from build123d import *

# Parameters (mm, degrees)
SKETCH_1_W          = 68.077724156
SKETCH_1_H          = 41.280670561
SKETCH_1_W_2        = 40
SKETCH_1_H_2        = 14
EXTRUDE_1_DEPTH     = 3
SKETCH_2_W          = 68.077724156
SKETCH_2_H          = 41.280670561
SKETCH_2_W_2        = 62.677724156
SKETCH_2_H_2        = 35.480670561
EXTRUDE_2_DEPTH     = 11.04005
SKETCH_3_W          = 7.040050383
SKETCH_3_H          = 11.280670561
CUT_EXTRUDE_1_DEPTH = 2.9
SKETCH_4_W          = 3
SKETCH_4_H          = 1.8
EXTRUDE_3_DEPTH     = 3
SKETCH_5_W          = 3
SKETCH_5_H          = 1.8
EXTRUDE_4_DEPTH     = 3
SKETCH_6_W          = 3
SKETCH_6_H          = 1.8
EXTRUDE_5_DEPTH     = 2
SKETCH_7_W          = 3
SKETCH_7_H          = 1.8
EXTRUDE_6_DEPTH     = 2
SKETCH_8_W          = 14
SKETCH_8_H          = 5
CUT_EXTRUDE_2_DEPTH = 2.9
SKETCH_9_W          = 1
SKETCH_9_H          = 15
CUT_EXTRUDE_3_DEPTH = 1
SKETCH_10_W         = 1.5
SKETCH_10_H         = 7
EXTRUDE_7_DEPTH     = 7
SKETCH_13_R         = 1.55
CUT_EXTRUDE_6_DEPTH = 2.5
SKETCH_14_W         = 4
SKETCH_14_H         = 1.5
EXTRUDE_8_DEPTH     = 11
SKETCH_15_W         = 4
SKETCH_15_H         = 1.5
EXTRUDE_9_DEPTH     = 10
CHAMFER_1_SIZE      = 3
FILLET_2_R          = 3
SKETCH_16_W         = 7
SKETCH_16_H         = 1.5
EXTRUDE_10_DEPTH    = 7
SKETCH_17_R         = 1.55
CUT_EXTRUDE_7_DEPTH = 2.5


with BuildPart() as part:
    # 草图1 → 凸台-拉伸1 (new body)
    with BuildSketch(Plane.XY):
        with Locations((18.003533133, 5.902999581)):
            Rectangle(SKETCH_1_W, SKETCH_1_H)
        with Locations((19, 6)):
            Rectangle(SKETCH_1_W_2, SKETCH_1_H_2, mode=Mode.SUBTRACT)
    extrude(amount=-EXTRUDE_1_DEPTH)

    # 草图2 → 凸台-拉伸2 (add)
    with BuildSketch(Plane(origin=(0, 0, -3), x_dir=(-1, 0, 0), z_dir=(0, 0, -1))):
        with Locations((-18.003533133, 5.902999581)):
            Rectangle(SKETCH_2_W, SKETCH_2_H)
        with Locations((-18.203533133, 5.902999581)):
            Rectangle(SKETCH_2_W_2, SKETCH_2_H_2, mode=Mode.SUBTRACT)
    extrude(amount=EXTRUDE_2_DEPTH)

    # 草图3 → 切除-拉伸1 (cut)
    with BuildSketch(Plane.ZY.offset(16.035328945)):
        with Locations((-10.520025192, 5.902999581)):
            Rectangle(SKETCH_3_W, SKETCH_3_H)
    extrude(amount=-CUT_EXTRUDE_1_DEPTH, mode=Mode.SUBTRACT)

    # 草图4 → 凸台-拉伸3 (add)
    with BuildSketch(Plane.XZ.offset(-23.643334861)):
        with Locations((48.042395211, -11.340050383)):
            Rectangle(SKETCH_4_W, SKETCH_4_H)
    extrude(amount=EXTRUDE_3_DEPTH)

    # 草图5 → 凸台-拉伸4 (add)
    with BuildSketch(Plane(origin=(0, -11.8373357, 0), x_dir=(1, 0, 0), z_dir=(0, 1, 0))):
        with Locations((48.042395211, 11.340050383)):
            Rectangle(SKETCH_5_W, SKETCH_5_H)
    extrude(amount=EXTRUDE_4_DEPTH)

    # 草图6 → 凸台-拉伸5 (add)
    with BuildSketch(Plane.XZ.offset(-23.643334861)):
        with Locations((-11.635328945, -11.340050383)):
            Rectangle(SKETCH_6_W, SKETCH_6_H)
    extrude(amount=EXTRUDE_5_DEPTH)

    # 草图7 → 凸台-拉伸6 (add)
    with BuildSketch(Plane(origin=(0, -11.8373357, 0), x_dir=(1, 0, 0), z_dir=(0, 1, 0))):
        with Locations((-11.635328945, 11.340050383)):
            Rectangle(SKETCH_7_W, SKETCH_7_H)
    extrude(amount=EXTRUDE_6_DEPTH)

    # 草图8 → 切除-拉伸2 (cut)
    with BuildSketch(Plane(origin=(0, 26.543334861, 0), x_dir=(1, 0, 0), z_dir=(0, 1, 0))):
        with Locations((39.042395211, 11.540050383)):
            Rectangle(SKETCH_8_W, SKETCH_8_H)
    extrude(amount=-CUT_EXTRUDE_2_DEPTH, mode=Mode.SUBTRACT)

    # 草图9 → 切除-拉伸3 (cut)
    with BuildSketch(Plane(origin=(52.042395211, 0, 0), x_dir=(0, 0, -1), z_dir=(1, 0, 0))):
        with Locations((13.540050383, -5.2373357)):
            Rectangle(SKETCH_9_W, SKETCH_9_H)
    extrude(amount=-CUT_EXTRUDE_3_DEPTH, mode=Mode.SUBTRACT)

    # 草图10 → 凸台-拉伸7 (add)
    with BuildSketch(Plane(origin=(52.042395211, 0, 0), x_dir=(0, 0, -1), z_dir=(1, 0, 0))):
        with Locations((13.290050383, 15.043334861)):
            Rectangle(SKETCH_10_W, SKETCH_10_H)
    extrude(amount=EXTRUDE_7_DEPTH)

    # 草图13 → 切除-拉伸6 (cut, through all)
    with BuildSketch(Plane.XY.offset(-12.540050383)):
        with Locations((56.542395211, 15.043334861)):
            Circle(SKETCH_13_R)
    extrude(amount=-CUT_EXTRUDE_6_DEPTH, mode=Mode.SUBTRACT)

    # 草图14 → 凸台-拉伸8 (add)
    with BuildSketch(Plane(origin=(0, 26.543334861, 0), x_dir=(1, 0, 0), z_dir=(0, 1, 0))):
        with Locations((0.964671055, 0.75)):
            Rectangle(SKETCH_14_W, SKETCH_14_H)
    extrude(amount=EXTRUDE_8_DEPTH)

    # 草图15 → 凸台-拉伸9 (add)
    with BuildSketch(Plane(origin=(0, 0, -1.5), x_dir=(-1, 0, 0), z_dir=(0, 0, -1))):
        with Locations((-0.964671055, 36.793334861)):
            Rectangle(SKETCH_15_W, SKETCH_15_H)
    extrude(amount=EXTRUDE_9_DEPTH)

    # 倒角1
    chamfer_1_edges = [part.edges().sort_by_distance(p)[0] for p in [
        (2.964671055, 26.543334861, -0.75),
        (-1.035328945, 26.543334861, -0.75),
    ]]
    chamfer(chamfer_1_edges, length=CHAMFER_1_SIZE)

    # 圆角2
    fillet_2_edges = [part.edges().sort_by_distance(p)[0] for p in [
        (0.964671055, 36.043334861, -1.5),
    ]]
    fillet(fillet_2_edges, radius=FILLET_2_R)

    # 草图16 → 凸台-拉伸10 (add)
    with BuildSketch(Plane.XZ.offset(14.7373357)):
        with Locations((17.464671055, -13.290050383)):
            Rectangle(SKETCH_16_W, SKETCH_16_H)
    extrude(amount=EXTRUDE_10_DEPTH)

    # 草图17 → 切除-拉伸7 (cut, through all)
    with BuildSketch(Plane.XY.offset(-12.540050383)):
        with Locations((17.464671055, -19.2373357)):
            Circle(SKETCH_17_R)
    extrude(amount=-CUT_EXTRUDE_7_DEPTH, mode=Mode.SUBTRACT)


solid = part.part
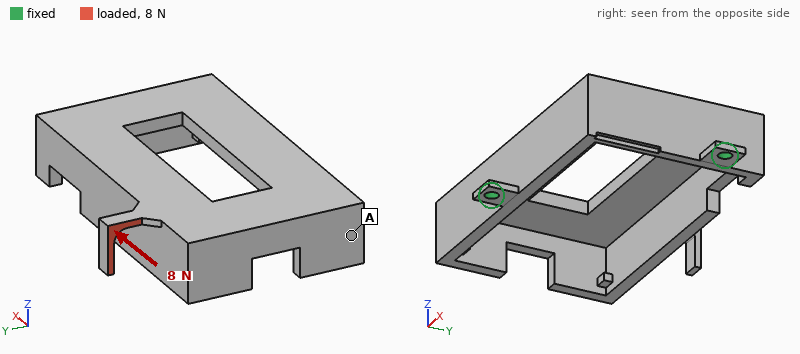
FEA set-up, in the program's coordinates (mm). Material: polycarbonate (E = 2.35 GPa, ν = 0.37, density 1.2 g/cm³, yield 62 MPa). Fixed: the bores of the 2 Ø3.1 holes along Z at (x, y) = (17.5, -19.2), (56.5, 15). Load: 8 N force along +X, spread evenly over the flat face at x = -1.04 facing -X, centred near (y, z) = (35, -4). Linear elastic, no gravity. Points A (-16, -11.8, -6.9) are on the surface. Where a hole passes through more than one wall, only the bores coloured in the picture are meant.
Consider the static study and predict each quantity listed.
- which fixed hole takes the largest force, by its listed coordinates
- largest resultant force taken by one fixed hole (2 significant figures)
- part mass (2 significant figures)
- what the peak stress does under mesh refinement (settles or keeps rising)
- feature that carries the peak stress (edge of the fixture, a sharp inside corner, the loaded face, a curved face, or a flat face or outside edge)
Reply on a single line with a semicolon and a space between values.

(56.5, 15); 9.3 N; 16 g; keeps rising; a sharp inside corner
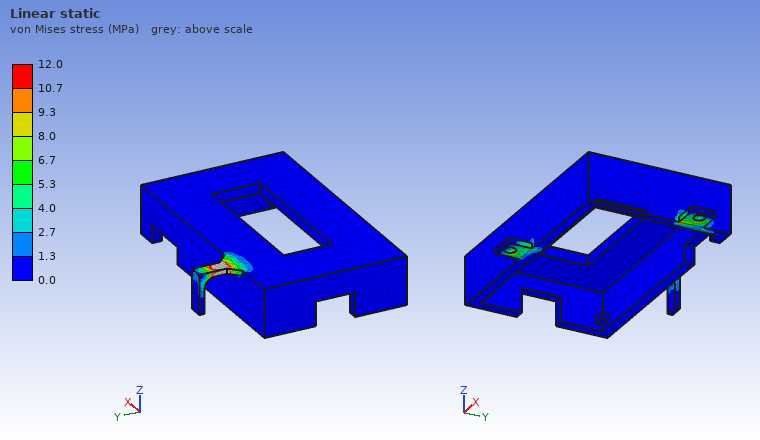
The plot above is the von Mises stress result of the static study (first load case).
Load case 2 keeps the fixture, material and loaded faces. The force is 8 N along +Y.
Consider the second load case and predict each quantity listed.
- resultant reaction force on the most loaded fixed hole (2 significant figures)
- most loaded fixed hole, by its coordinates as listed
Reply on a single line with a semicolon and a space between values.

8.8 N; (17.5, -19.2)
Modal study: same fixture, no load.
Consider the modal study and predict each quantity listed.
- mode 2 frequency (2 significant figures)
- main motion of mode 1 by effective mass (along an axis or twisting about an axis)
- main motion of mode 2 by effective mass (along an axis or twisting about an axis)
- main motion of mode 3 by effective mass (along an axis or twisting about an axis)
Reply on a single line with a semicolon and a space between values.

440 Hz; along Z; along Y; along X
